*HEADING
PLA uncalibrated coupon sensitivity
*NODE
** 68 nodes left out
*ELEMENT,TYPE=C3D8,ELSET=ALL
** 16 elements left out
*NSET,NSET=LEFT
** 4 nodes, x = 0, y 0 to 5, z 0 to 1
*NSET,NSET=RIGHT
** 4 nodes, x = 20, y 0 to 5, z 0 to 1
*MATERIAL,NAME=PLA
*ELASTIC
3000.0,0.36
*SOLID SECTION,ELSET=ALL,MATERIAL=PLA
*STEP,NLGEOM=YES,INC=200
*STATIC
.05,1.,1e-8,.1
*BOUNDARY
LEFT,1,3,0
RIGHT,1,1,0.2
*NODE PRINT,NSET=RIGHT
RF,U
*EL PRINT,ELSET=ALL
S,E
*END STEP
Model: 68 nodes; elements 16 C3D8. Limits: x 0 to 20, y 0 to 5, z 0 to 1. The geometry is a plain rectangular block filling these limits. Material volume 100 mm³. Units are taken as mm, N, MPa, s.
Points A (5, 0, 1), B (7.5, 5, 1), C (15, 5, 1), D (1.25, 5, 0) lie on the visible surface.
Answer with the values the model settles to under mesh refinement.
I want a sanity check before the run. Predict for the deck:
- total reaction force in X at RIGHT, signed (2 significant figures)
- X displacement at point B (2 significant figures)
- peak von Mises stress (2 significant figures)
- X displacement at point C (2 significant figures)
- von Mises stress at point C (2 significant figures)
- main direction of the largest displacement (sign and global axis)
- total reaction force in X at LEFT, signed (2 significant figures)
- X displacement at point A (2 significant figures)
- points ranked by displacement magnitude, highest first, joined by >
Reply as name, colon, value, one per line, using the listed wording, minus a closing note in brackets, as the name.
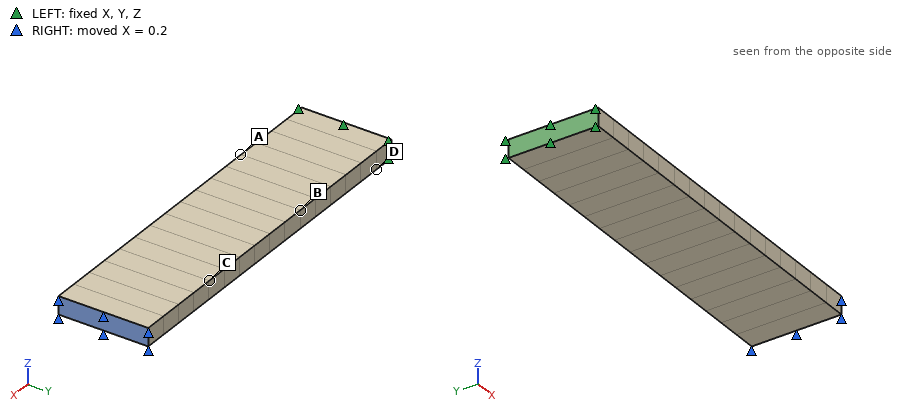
total reaction force in X at RIGHT, signed: 150 N
X displacement at point B: 0.074 mm
peak von Mises stress: 32 MPa
X displacement at point C: 0.15 mm
von Mises stress at point C: 31 MPa
main direction of the largest displacement: +X
total reaction force in X at LEFT, signed: -150 N
X displacement at point A: 0.049 mm
points ranked by displacement magnitude, highest first, joined by >: C > B > A > D
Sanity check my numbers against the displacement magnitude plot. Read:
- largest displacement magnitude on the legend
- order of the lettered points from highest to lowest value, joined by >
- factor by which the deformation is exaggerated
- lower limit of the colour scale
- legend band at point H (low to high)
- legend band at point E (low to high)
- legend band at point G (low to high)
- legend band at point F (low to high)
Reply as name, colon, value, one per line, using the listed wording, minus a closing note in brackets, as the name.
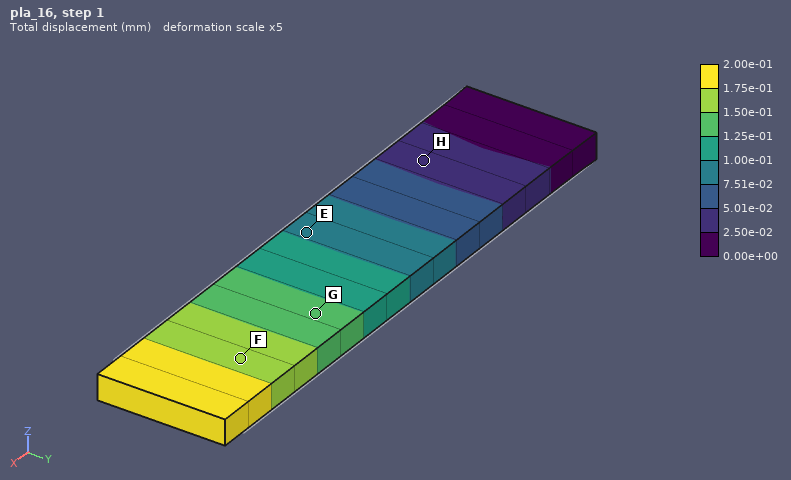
largest displacement magnitude on the legend: 2.00e-01 mm
order of the lettered points from highest to lowest value, joined by >: F > G > E > H
factor by which the deformation is exaggerated: 5
lower limit of the colour scale: 0.00e+00 mm
legend band at point H: 2.50e-02 to 5.01e-02 mm
legend band at point E: 7.51e-02 to 1.00e-01 mm
legend band at point G: 1.25e-01 to 1.50e-01 mm
legend band at point F: 1.50e-01 to 1.75e-01 mm
